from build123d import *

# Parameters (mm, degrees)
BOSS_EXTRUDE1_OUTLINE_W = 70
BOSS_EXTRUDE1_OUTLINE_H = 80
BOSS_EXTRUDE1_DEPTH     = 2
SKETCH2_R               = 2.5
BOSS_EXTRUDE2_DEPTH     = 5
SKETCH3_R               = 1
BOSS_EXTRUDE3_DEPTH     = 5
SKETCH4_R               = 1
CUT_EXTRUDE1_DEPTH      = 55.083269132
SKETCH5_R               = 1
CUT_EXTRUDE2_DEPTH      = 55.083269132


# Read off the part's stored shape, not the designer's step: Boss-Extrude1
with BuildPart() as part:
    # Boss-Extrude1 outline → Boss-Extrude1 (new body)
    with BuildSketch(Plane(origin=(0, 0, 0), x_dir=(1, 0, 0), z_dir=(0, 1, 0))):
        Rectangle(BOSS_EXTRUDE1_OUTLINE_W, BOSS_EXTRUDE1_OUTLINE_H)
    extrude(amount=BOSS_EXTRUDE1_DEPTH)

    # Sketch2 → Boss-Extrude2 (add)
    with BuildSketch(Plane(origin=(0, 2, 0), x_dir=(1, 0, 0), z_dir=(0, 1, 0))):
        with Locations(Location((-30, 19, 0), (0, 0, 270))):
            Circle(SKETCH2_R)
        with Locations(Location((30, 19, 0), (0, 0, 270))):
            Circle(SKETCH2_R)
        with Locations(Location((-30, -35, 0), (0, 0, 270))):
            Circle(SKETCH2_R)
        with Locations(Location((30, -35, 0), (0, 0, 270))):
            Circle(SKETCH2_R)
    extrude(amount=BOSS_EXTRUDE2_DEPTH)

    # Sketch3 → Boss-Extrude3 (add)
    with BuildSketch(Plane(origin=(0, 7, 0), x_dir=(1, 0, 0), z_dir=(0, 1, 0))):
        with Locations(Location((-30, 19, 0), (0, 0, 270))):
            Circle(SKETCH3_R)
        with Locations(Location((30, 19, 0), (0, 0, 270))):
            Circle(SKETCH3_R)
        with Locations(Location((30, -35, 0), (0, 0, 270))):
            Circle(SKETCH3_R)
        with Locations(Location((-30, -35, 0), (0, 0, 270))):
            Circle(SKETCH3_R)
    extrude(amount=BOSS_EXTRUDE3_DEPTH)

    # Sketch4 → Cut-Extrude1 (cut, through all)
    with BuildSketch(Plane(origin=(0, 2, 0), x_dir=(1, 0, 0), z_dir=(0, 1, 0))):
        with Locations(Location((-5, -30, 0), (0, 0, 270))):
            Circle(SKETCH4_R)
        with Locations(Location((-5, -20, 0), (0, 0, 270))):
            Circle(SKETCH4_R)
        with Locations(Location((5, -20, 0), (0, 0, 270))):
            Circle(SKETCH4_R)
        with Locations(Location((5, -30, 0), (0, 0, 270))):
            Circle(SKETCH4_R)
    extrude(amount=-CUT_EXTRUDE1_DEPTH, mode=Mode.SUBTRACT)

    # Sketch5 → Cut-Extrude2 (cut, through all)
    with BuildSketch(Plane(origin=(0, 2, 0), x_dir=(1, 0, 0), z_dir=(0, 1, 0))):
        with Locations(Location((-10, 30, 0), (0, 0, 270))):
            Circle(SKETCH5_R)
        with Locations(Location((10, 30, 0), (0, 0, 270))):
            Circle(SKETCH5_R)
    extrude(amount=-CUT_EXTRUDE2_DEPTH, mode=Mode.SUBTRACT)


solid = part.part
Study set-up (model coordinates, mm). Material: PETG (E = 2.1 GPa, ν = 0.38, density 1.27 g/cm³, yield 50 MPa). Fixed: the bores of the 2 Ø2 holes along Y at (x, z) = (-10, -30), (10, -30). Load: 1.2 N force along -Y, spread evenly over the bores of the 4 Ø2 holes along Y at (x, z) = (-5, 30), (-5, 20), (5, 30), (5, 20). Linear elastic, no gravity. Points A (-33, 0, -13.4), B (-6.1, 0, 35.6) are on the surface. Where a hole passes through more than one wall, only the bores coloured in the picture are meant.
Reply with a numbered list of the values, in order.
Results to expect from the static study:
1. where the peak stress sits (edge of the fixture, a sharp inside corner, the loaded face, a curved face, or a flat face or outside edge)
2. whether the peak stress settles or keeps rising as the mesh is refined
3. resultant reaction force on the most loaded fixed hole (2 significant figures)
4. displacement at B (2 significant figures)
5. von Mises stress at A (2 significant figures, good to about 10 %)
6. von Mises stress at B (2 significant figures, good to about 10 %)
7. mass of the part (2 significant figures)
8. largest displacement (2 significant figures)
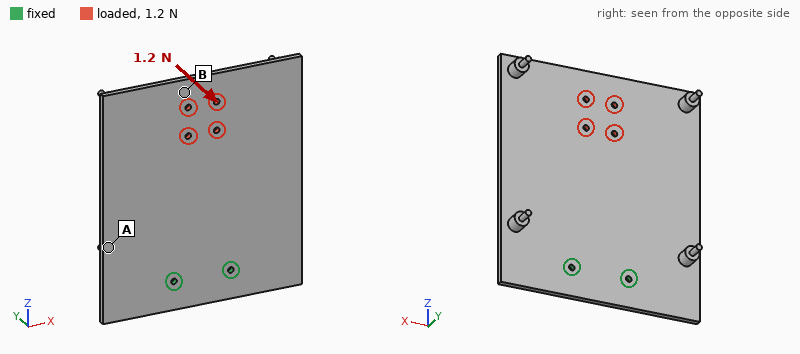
1. edge of the fixture
2. keeps rising
3. 0.60 N
4. 1.1 mm
5. 0.86 MPa
6. 0.31 MPa
7. 15 g
8. 1.2 mm
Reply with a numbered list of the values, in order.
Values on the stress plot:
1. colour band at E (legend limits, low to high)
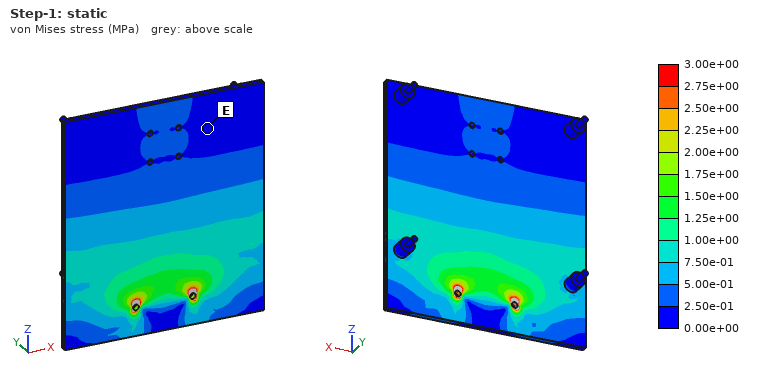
1. 0.00e+00 to 2.50e-01 MPa
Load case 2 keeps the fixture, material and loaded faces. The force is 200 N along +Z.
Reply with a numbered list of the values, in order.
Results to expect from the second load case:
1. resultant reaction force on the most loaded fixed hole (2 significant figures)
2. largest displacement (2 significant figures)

1. 100 N
2. 83 µm
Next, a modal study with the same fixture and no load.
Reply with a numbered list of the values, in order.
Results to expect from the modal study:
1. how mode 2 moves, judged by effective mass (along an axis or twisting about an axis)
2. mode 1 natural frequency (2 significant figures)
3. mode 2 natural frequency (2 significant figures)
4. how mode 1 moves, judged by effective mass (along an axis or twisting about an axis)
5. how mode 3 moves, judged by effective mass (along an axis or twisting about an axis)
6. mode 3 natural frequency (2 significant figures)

1. twisting about Z
2. 75 Hz
3. 160 Hz
4. along Y
5. along Y
6. 410 Hz
